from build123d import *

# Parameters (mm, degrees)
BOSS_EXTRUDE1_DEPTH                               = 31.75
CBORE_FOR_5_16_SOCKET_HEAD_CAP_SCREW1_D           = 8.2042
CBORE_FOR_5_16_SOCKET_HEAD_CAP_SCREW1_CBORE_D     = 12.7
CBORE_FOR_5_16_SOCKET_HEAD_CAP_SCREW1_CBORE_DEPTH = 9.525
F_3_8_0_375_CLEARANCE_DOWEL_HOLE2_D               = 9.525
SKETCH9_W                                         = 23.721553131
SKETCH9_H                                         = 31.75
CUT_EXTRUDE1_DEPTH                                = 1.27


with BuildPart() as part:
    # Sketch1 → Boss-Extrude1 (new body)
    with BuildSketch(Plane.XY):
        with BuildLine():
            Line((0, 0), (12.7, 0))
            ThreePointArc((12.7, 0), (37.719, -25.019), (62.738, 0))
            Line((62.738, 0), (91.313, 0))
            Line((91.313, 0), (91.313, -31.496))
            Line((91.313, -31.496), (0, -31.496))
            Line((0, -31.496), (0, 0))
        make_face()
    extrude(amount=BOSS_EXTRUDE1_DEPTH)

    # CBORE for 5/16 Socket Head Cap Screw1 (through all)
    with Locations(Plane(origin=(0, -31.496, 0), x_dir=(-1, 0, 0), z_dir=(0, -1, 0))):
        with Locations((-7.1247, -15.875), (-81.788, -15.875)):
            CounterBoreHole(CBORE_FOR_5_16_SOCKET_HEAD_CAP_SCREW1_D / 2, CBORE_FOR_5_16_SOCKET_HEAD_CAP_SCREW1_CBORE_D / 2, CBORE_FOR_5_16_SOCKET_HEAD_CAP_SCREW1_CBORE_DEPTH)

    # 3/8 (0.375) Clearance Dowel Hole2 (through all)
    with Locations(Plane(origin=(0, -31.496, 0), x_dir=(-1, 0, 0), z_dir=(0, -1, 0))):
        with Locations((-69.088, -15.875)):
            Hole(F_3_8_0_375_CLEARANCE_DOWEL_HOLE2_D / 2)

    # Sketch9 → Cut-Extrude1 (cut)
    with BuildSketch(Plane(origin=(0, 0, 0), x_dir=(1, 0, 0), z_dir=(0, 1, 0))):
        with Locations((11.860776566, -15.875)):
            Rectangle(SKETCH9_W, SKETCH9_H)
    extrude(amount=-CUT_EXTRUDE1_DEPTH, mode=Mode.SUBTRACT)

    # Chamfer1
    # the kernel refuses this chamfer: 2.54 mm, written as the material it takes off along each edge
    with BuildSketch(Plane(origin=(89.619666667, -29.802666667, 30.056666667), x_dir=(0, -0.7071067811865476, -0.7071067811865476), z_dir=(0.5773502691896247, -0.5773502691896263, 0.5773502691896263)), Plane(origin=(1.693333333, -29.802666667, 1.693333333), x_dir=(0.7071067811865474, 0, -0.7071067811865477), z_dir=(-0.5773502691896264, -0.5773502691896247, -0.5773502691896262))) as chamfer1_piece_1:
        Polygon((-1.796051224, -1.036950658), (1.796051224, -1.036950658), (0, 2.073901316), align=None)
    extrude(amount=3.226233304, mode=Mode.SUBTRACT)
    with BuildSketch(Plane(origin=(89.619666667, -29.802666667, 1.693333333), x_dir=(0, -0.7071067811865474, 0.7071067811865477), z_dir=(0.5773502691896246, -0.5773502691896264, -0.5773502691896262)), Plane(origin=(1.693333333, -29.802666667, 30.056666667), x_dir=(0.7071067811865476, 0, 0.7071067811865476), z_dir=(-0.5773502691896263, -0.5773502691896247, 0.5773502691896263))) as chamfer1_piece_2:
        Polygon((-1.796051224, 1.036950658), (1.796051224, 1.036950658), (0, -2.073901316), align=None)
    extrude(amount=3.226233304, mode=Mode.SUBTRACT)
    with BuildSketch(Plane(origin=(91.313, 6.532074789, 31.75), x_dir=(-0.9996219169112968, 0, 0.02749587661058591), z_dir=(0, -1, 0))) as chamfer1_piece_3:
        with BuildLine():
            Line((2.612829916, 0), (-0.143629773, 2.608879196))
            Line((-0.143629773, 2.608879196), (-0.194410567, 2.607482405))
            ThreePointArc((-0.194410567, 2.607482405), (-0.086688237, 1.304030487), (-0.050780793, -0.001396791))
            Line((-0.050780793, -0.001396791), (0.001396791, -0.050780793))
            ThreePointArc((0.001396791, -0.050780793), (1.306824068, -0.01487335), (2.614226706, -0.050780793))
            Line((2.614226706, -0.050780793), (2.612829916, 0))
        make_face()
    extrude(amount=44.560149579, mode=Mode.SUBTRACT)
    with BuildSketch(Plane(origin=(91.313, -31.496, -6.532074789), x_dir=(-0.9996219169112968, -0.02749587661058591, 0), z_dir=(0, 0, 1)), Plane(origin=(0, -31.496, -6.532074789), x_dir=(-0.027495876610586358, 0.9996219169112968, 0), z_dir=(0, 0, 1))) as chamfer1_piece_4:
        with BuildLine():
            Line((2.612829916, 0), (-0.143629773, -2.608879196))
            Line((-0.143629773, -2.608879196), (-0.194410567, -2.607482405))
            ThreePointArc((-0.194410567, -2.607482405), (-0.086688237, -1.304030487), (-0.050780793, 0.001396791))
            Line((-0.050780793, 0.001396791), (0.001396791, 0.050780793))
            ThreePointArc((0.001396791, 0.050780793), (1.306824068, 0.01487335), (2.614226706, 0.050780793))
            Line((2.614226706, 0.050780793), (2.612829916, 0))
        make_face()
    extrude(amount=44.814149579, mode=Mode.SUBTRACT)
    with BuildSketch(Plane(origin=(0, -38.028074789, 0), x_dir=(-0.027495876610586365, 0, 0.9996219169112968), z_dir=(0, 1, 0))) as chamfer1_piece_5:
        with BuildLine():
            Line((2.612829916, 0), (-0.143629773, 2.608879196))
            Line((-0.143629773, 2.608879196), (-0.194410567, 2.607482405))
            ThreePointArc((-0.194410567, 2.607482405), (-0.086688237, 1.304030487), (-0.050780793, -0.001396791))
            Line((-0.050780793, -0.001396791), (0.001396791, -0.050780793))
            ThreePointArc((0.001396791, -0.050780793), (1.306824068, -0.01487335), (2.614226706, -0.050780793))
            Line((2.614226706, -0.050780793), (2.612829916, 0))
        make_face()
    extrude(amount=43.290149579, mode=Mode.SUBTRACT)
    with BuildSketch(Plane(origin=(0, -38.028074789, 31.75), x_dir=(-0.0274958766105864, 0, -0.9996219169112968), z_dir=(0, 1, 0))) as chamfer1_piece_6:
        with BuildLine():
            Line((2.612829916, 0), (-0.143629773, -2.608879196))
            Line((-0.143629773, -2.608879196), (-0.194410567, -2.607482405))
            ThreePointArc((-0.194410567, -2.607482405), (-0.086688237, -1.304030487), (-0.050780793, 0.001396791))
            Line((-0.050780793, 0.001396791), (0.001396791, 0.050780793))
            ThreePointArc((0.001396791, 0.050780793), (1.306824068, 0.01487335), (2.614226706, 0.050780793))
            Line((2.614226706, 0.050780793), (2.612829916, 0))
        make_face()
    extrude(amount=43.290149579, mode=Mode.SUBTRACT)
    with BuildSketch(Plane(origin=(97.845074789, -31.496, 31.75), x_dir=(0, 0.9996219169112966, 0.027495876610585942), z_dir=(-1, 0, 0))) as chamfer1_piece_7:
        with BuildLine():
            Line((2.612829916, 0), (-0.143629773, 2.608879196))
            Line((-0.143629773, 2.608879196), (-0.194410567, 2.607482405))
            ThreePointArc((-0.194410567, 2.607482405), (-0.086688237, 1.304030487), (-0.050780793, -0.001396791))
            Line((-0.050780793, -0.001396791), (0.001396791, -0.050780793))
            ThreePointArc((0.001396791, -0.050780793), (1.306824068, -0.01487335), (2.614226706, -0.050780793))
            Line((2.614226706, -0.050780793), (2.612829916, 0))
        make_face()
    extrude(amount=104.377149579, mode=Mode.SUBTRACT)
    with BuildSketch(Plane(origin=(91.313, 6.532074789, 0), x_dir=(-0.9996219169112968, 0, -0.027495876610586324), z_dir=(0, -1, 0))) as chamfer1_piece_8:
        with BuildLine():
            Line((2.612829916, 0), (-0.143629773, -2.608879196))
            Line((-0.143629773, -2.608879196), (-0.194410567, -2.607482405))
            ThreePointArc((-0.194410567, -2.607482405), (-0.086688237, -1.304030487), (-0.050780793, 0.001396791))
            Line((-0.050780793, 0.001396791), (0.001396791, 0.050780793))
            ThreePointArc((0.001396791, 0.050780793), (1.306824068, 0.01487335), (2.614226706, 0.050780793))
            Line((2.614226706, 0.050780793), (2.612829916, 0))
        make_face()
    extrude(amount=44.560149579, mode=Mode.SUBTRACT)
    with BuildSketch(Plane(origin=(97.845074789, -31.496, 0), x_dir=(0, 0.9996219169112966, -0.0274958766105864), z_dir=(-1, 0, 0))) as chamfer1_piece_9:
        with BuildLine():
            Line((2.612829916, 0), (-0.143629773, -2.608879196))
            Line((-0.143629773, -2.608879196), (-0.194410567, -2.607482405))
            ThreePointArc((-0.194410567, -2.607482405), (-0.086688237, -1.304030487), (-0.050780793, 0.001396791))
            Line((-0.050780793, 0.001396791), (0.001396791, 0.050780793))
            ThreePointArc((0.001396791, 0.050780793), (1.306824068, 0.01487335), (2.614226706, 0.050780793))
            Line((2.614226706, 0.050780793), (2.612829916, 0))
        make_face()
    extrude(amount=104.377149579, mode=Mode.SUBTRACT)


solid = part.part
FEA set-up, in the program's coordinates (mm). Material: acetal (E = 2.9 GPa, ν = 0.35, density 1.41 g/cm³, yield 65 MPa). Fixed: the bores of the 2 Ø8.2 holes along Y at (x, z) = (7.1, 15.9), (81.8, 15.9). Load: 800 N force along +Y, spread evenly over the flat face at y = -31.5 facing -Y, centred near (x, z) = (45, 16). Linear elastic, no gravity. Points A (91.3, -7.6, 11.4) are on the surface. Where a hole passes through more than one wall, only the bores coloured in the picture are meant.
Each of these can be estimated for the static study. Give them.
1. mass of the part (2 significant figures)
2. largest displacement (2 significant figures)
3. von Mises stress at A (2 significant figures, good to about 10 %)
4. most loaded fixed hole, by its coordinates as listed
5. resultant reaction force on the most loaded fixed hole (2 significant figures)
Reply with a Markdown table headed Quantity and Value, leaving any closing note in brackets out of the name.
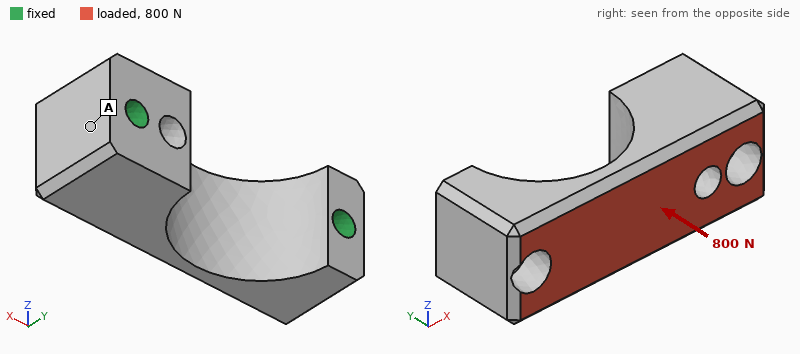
| Quantity | Value |
|---|---|
| mass of the part | 73 g |
| largest displacement | 42 µm |
| von Mises stress at A | 0.68 MPa |
| most loaded fixed hole, by its coordinates as listed | (81.8, 15.9) |
| resultant reaction force on the most loaded fixed hole | 510 N |
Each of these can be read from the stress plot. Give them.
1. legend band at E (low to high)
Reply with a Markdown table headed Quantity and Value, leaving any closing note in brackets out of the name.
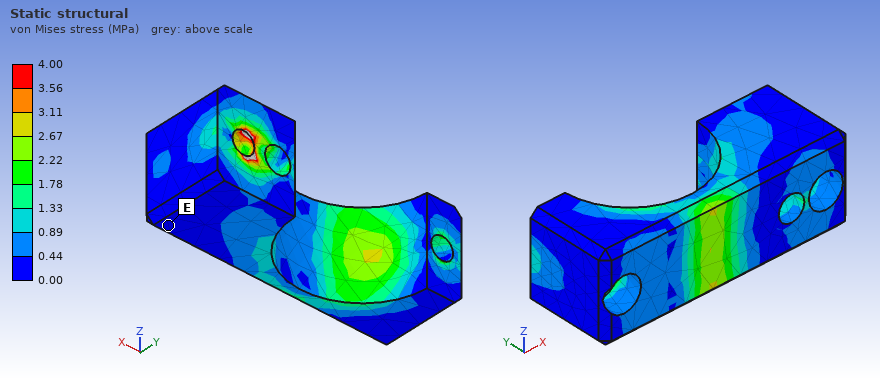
| Quantity | Value |
|---|---|
| legend band at E | 0.00 to 0.44 MPa |
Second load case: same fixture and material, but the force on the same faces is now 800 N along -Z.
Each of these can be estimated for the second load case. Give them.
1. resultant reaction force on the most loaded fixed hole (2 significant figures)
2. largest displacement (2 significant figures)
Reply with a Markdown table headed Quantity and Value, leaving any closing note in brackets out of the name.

| Quantity | Value |
|---|---|
| resultant reaction force on the most loaded fixed hole | 410 N |
| largest displacement | 88 µm |
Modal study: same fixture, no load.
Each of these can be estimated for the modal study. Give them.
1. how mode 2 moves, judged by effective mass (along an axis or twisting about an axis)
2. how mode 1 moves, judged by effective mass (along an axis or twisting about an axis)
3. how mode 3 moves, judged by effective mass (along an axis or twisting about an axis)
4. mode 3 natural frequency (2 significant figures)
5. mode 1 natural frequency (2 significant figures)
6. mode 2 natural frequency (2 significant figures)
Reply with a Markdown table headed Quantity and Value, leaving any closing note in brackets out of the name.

| Quantity | Value |
|---|---|
| how mode 2 moves, judged by effective mass | along Y |
| how mode 1 moves, judged by effective mass | along Z |
| how mode 3 moves, judged by effective mass | along X |
| mode 3 natural frequency | 5400 Hz |
| mode 1 natural frequency | 3300 Hz |
| mode 2 natural frequency | 4100 Hz |
